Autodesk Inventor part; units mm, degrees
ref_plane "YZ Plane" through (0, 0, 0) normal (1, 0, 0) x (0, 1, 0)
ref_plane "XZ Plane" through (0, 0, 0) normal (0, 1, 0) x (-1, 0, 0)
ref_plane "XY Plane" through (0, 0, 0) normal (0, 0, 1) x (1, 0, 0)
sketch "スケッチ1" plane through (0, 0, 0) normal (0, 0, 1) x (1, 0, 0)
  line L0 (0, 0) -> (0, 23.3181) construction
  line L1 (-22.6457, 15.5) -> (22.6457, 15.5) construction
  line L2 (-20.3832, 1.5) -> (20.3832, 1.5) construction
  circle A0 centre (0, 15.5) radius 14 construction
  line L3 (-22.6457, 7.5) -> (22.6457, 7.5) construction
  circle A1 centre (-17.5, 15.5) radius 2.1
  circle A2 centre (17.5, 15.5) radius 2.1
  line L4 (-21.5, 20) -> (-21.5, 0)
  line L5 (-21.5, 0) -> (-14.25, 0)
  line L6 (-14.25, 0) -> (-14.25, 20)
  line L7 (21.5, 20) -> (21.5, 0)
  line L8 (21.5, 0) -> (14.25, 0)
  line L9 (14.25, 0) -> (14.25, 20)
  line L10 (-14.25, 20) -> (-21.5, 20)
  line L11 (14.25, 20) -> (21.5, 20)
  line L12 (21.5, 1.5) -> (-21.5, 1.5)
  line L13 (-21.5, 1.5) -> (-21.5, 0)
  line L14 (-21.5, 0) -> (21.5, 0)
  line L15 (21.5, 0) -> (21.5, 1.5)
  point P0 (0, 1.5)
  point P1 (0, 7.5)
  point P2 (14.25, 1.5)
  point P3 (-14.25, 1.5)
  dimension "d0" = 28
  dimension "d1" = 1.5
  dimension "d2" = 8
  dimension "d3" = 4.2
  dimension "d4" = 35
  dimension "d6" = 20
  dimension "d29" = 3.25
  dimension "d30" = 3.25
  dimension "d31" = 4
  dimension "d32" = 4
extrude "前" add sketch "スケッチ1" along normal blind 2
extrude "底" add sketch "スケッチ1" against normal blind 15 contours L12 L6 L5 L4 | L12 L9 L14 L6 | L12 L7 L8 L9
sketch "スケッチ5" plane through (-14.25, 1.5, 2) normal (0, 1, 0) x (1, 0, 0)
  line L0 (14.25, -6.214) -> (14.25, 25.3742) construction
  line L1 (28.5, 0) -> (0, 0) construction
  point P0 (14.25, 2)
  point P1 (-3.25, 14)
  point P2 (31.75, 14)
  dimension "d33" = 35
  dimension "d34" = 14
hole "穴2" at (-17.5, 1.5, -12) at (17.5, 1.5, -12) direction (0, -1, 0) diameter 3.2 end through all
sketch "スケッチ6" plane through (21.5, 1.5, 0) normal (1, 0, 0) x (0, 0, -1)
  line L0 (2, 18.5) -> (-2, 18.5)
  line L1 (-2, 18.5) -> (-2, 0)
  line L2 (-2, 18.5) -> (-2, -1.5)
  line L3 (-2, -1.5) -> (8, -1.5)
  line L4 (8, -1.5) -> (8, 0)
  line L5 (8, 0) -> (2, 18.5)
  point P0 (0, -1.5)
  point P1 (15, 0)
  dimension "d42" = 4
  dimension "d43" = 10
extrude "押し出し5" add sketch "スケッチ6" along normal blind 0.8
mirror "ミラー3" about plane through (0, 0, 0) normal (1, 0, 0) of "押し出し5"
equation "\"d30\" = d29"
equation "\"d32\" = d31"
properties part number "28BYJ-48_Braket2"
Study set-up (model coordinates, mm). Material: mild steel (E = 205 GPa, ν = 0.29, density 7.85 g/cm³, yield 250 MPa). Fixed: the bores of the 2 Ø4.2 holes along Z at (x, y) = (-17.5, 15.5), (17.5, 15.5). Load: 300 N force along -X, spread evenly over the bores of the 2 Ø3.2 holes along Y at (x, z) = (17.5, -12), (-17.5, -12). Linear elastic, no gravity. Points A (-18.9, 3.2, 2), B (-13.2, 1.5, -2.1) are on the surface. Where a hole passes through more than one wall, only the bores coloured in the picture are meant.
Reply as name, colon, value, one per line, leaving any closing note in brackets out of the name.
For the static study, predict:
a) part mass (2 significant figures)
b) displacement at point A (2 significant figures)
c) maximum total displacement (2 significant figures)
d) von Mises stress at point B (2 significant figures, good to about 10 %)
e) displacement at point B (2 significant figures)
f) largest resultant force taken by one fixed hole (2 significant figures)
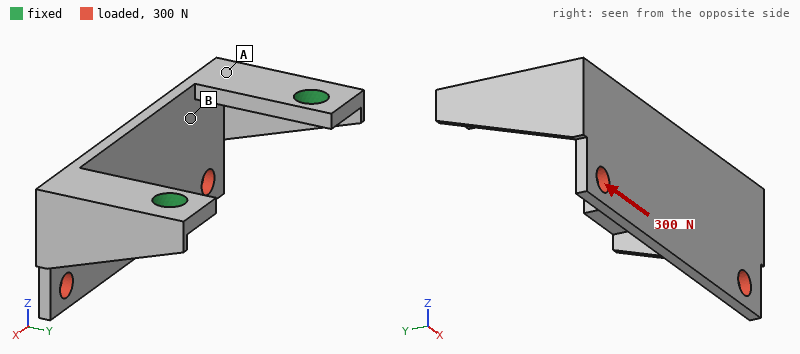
part mass: 14 g
displacement at point A: 22 µm
maximum total displacement: 54 µm
von Mises stress at point B: 48 MPa
displacement at point B: 24 µm
largest resultant force taken by one fixed hole: 180 N
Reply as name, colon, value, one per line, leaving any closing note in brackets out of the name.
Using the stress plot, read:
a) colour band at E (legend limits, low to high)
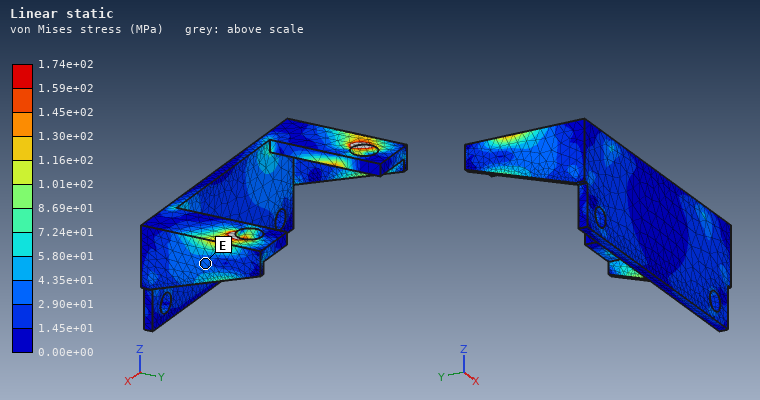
colour band at E: 2.90e+01 to 4.35e+01 MPa
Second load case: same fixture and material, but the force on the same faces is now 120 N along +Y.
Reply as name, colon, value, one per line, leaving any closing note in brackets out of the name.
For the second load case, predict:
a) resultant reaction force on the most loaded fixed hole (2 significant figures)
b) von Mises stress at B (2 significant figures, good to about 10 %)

resultant reaction force on the most loaded fixed hole: 66 N
von Mises stress at B: 38 MPa
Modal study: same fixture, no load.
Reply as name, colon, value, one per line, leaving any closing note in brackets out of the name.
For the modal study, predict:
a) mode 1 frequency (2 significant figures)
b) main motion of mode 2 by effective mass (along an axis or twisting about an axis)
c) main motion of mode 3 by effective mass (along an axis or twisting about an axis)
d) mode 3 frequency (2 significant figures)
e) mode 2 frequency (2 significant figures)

mode 1 frequency: 2800 Hz
main motion of mode 2 by effective mass: along X
main motion of mode 3 by effective mass: along Z
mode 3 frequency: 5100 Hz
mode 2 frequency: 4700 Hz
